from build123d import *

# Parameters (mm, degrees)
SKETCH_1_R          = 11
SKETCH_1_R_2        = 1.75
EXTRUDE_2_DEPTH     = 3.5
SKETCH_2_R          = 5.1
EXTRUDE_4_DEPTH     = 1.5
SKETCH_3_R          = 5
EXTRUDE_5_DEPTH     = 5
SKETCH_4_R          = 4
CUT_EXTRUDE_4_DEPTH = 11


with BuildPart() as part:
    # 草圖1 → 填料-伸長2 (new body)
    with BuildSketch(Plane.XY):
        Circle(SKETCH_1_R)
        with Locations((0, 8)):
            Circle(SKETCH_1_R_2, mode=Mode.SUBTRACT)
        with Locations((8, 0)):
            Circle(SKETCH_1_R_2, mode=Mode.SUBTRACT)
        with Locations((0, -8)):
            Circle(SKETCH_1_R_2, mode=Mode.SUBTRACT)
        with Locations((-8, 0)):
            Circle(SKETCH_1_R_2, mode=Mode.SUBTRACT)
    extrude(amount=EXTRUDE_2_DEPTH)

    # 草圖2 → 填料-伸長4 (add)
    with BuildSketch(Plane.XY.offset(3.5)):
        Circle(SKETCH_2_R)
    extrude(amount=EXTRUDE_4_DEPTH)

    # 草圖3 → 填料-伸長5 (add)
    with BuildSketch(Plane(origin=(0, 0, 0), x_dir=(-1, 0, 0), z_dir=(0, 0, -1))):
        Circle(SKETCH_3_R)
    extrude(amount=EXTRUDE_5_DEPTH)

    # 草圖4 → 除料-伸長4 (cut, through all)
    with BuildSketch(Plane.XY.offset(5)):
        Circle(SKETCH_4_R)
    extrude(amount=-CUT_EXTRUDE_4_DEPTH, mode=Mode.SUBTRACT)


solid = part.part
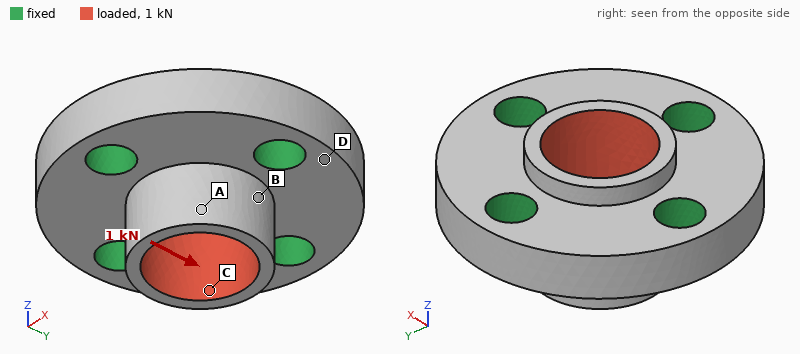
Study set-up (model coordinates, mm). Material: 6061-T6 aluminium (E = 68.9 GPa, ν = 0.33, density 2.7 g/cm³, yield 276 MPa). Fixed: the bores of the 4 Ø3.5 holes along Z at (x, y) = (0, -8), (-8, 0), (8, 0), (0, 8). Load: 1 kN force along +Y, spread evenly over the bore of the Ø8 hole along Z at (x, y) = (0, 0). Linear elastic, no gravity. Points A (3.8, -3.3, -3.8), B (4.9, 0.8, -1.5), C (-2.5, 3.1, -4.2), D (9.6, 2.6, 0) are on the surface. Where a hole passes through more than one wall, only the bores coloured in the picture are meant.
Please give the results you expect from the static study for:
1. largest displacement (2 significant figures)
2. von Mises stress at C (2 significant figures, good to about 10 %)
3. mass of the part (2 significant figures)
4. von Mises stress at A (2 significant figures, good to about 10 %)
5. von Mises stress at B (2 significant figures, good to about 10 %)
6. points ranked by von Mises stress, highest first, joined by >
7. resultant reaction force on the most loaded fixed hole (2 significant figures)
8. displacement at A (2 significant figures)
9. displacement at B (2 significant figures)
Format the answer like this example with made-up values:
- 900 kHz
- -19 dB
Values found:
- 6.9 µm
- 20 MPa
- 3.3 g
- 15 MPa
- 29 MPa
- B > C > A > D
- 310 N
- 5.2 µm
- 2.8 µm
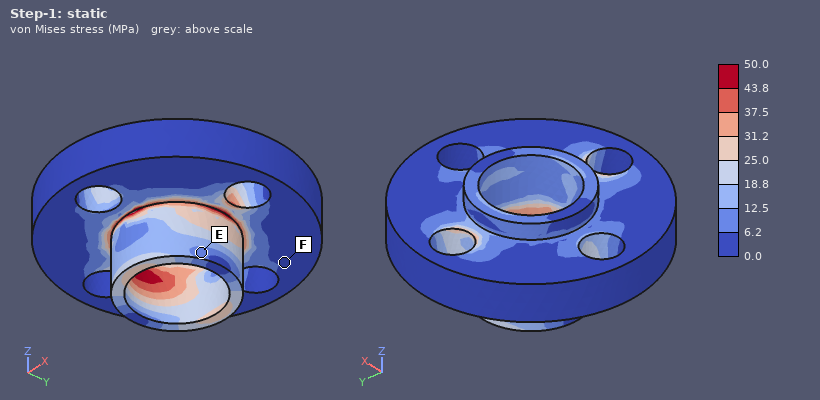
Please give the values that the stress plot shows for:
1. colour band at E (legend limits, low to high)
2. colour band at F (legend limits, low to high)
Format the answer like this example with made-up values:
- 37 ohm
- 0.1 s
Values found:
- 6.2 to 12.5 MPa
- 0.0 to 6.2 MPa
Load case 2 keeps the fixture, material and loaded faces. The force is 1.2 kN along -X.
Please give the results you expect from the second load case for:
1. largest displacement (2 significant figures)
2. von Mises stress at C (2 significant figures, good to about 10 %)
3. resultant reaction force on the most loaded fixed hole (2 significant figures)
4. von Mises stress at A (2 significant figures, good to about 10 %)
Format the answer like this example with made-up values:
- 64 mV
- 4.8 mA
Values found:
- 8.3 µm
- 23 MPa
- 370 N
- 19 MPa
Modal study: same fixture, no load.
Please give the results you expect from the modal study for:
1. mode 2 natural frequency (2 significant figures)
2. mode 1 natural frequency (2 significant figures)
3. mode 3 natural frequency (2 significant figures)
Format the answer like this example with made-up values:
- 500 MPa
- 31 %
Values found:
- 71 kHz
- 67 kHz
- 82 kHz
